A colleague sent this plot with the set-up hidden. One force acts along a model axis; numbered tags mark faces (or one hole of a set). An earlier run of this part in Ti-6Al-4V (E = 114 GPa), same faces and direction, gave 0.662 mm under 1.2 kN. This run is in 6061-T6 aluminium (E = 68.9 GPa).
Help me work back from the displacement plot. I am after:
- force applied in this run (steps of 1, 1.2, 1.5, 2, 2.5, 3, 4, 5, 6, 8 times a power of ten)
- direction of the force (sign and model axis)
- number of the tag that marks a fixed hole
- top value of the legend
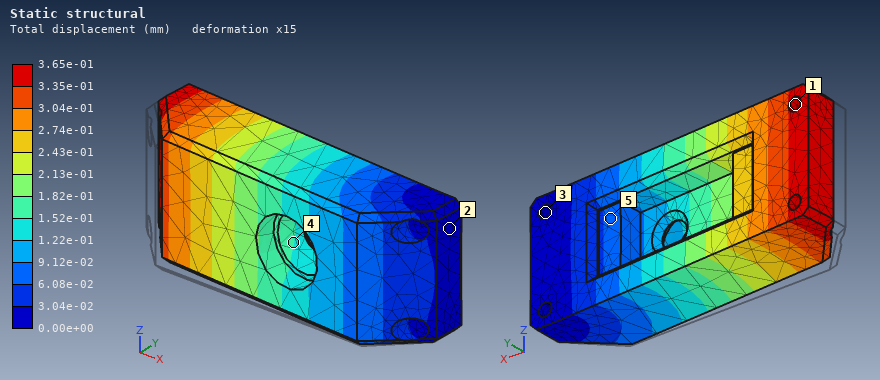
400 N
+Y
3
3.65e-01 mm
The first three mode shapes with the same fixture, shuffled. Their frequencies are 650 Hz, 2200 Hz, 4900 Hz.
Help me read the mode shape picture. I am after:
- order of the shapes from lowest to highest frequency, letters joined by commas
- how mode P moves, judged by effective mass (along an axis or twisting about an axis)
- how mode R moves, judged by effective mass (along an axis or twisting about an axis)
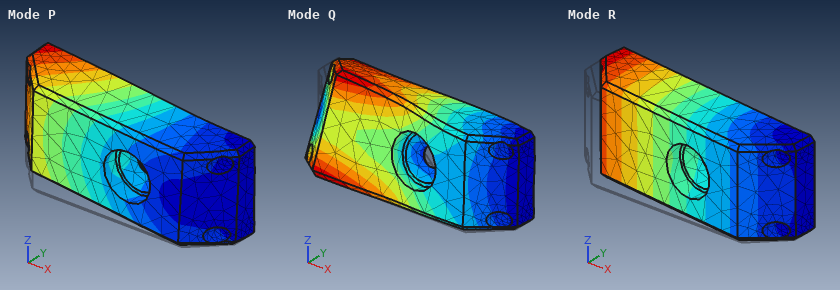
R, P, Q
along Z
along Y
